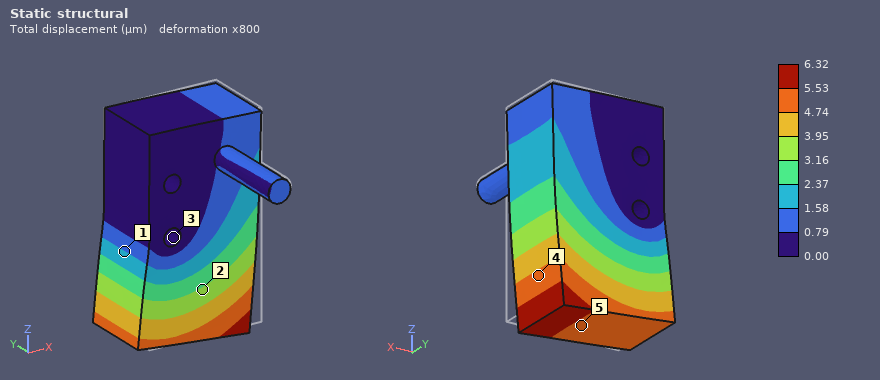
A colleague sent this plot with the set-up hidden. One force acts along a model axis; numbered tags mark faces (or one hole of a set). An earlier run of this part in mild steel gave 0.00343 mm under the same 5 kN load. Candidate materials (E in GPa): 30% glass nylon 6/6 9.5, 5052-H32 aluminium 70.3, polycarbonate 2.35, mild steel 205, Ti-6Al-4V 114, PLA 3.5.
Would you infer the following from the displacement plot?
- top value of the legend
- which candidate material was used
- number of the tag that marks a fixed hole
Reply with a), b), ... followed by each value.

a) 6.32 µm
b) Ti-6Al-4V
c) 3
